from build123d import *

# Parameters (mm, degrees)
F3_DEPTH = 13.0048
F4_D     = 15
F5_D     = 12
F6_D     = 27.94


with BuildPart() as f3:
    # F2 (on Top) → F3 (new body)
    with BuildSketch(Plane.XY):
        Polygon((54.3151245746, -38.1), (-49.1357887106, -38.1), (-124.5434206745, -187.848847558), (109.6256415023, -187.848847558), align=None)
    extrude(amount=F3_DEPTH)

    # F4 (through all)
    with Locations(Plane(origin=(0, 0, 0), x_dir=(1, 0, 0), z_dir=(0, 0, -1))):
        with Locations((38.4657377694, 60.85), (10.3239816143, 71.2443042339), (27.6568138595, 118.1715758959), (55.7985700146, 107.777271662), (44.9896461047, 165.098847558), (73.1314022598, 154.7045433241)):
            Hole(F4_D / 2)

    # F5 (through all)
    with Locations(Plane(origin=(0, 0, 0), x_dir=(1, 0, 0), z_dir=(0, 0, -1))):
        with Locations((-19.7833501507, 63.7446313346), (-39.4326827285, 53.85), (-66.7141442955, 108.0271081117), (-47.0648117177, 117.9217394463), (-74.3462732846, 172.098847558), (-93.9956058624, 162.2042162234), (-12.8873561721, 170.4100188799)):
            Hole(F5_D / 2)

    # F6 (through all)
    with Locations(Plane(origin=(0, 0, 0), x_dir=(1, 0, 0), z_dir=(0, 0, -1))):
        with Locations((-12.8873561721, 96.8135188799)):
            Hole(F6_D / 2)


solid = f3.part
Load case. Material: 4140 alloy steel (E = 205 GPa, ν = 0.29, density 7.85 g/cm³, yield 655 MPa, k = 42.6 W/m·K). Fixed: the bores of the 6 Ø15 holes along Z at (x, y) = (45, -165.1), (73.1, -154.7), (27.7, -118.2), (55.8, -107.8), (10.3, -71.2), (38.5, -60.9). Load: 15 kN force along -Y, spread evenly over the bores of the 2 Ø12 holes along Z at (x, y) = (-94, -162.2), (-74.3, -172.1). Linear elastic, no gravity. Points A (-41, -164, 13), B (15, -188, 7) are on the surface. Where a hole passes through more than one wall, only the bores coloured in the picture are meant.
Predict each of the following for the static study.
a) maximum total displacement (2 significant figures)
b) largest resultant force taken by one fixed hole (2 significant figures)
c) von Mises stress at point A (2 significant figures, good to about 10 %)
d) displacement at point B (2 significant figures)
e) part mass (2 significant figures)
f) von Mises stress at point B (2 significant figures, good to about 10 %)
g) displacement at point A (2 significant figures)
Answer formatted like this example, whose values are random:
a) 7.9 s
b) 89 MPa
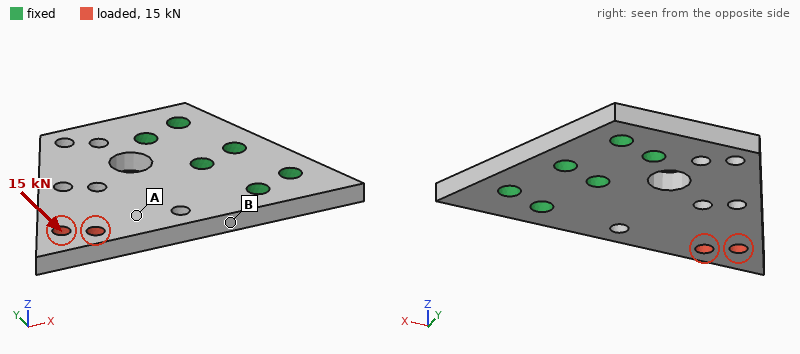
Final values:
a) 51 µm
b) 13 kN
c) 14 MPa
d) 7.7 µm
e) 2.3 kg
f) 35 MPa
g) 19 µm
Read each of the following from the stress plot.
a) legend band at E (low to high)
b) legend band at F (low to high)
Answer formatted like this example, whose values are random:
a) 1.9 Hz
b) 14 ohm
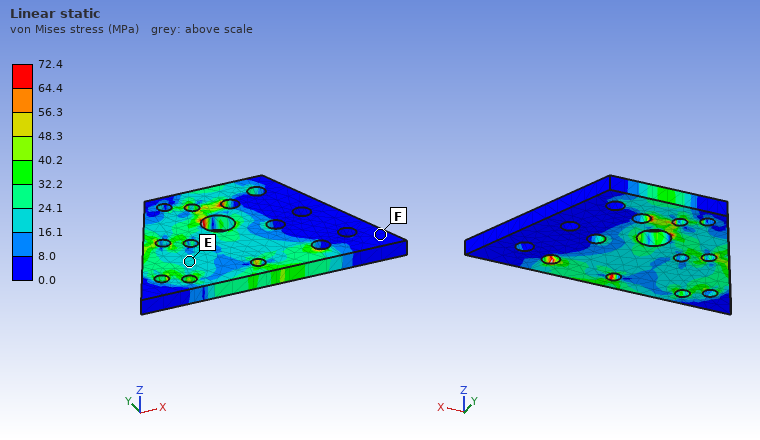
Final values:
a) 16.1 to 24.1 MPa
b) 0.0 to 8.0 MPa
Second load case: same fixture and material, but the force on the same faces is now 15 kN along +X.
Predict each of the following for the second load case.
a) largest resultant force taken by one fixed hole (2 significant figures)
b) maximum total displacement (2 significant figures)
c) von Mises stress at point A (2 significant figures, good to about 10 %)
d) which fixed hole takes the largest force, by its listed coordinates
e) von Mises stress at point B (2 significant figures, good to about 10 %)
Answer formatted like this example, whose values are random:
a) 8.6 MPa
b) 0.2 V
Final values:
a) 9.9 kN
b) 26 µm
c) 20 MPa
d) (45, -165.1)
e) 24 MPa
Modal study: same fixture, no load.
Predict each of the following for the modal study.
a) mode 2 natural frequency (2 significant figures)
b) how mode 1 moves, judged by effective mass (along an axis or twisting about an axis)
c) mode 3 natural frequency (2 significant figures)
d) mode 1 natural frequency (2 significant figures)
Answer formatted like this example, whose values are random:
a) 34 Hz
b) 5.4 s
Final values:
a) 2100 Hz
b) along Z
c) 3200 Hz
d) 690 Hz
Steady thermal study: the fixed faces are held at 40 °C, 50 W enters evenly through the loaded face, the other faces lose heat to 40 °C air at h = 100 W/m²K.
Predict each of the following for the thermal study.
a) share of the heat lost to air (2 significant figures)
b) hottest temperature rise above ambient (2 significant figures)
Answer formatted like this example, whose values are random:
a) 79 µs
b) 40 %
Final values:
a) 88 %
b) 49 K
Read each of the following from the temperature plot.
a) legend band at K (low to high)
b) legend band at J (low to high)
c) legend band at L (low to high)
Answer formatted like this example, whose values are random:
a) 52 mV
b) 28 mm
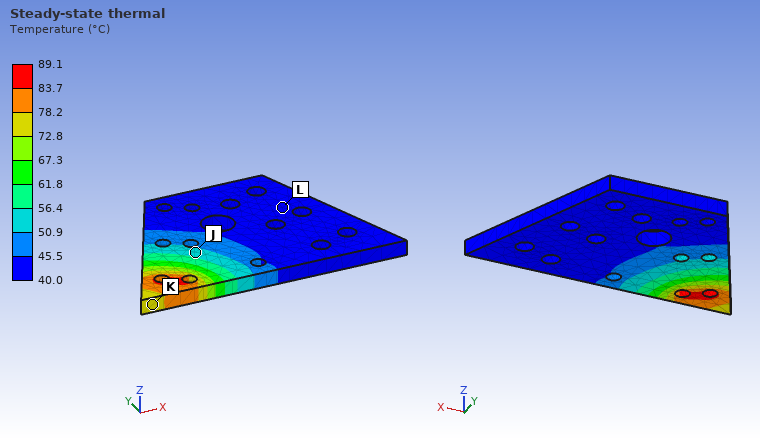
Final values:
a) 72.8 to 78.2 °C
b) 50.9 to 56.4 °C
c) 40.0 to 45.5 °C
